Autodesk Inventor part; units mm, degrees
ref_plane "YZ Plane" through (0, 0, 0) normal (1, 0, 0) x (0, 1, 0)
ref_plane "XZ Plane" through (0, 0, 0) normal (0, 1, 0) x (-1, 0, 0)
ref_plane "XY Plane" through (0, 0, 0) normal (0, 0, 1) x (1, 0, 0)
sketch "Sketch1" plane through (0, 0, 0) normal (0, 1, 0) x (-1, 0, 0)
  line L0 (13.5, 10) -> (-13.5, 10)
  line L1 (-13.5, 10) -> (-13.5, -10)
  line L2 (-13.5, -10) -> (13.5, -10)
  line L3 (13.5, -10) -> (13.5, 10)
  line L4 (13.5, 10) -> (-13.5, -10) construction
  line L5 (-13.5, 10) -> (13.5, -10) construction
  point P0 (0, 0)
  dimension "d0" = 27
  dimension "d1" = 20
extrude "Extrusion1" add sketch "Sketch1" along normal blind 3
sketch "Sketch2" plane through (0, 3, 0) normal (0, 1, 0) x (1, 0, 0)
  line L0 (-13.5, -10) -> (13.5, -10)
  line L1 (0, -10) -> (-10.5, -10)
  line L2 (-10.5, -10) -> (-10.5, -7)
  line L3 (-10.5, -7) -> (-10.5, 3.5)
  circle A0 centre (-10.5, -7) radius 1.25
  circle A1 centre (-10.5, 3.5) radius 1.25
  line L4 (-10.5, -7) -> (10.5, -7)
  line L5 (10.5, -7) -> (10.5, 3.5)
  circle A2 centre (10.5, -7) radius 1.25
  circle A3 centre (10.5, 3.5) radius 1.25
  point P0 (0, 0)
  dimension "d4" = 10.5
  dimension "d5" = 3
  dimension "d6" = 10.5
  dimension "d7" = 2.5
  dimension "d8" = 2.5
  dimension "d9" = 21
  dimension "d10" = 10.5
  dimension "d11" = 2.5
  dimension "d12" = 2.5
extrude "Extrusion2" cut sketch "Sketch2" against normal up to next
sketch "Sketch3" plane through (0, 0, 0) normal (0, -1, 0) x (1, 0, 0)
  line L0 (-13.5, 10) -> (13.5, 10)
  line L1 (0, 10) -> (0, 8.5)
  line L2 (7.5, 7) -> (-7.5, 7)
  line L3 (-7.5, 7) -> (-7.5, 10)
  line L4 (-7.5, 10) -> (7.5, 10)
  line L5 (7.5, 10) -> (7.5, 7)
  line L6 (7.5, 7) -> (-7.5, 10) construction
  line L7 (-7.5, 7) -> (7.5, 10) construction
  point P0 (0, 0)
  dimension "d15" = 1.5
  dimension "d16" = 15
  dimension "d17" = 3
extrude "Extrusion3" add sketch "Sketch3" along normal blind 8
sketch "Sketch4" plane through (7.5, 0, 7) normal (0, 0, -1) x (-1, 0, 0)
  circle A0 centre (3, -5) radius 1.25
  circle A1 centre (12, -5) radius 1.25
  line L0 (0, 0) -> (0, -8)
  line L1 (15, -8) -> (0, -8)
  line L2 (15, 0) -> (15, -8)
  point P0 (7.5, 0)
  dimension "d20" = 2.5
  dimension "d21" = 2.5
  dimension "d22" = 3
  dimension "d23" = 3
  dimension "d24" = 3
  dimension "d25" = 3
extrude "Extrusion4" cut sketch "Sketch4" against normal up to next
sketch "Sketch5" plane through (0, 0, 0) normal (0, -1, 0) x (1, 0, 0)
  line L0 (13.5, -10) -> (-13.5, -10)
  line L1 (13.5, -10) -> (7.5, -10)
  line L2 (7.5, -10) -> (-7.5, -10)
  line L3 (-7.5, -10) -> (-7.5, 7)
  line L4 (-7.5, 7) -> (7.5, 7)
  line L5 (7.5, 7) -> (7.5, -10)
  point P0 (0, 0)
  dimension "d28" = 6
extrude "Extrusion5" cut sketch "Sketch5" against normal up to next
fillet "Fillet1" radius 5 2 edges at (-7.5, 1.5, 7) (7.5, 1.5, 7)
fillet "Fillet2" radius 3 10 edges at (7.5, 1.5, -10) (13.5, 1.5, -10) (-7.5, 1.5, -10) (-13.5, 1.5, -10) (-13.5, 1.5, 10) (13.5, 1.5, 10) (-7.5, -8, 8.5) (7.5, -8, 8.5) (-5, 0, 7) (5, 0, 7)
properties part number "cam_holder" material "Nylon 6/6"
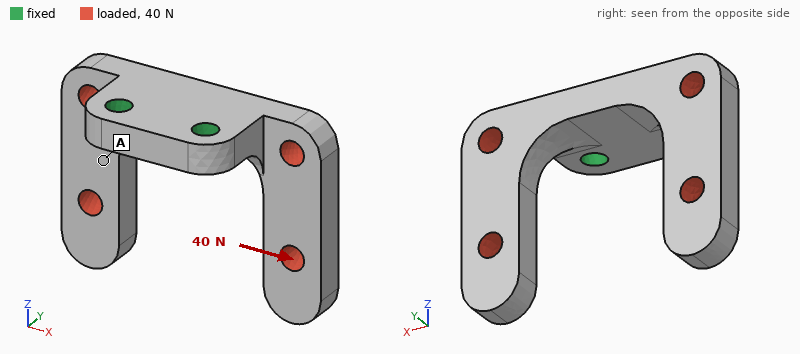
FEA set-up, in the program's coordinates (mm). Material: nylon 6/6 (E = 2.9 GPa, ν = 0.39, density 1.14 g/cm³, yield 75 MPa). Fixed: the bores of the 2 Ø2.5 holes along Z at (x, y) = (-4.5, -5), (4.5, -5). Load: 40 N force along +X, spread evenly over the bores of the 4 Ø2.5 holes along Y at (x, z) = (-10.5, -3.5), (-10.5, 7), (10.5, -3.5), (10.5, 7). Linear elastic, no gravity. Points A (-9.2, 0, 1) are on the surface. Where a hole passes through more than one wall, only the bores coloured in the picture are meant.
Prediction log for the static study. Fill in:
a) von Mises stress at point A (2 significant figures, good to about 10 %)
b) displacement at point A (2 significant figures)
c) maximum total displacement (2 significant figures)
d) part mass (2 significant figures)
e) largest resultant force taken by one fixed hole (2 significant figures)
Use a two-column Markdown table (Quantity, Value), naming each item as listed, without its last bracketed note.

| Quantity | Value |
|---|---|
| von Mises stress at point A | 1.6 MPa |
| displacement at point A | 0.14 mm |
| maximum total displacement | 0.35 mm |
| part mass | 1.3 g |
| largest resultant force taken by one fixed hole | 35 N |
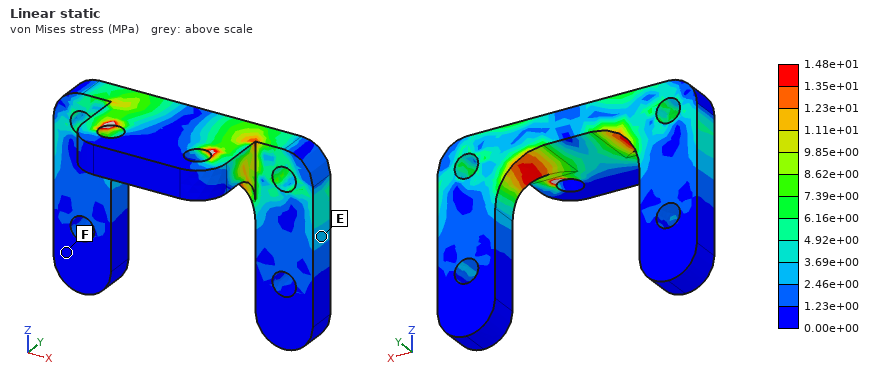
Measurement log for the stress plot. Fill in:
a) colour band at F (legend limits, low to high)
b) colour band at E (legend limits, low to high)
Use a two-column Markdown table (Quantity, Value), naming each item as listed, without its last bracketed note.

| Quantity | Value |
|---|---|
| colour band at F | 0.00e+00 to 1.23e+00 MPa |
| colour band at E | 2.46e+00 to 3.69e+00 MPa |
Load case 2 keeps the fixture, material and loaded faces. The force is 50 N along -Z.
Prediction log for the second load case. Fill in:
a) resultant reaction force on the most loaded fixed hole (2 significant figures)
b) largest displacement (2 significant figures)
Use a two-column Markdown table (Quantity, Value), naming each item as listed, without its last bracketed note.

| Quantity | Value |
|---|---|
| resultant reaction force on the most loaded fixed hole | 25 N |
| largest displacement | 0.36 mm |
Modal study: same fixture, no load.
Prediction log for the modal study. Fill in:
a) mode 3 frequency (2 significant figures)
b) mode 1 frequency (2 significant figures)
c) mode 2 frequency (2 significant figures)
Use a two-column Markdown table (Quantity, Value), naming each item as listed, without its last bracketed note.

| Quantity | Value |
|---|---|
| mode 3 frequency | 2000 Hz |
| mode 1 frequency | 1700 Hz |
| mode 2 frequency | 1700 Hz |
